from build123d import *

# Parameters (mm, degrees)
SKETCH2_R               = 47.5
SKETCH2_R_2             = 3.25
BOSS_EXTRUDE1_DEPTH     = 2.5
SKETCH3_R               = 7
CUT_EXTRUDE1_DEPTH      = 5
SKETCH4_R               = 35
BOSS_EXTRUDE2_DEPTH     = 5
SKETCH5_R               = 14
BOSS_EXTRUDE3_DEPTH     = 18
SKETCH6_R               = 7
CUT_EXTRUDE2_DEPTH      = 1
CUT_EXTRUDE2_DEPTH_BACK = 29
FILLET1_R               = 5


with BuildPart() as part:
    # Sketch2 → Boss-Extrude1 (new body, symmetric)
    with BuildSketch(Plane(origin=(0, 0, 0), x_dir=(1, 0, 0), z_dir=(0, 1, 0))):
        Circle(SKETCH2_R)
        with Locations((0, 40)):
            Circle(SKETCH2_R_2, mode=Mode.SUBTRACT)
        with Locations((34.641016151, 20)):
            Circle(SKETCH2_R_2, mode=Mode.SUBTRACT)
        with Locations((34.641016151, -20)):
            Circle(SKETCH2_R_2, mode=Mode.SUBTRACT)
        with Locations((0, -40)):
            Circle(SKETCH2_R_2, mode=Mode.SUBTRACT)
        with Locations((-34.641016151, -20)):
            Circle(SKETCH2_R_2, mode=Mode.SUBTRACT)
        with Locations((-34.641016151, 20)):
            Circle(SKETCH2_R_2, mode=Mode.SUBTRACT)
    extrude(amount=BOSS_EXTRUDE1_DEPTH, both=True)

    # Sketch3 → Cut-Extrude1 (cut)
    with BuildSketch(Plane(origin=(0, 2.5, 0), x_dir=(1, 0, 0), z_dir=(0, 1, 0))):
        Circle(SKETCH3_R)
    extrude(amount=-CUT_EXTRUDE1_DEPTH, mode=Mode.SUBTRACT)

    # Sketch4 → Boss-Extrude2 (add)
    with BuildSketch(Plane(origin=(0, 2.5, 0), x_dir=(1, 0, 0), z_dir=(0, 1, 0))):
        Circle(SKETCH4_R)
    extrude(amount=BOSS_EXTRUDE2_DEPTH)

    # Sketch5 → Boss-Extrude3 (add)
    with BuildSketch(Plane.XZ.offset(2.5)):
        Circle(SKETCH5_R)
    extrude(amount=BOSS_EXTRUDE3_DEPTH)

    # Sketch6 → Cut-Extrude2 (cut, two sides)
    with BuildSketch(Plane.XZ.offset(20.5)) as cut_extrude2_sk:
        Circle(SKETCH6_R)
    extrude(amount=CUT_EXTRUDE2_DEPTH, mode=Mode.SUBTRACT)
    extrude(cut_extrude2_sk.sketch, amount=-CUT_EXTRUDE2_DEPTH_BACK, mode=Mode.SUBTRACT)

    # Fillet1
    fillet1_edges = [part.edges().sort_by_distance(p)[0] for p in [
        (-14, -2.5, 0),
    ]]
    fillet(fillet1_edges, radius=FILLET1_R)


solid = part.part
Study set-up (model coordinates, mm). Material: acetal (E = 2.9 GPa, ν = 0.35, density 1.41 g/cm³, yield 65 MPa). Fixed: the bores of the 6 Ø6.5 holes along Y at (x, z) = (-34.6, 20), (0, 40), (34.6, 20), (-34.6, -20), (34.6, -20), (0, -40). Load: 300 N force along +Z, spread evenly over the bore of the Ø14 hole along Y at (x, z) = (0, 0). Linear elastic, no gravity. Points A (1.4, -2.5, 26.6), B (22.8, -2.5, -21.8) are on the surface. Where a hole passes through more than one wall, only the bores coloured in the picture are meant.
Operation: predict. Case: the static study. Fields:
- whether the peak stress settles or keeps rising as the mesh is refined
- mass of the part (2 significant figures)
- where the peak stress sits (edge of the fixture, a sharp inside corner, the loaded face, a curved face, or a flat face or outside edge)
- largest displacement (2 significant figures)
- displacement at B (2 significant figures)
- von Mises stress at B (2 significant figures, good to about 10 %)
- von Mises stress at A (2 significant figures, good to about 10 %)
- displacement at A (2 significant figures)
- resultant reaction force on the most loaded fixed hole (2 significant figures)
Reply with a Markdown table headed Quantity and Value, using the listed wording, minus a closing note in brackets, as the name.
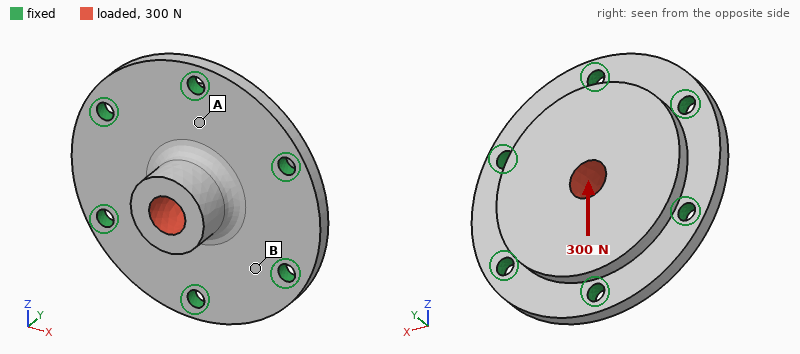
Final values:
| Quantity | Value |
|---|---|
| whether the peak stress settles or keeps rising as the mesh is refined | keeps rising |
| mass of the part | 86 g |
| where the peak stress sits | edge of the fixture |
| largest displacement | 25 µm |
| displacement at B | 4.0 µm |
| von Mises stress at B | 0.27 MPa |
| von Mises stress at A | 0.95 MPa |
| displacement at A | 6.1 µm |
| resultant reaction force on the most loaded fixed hole | 70 N |
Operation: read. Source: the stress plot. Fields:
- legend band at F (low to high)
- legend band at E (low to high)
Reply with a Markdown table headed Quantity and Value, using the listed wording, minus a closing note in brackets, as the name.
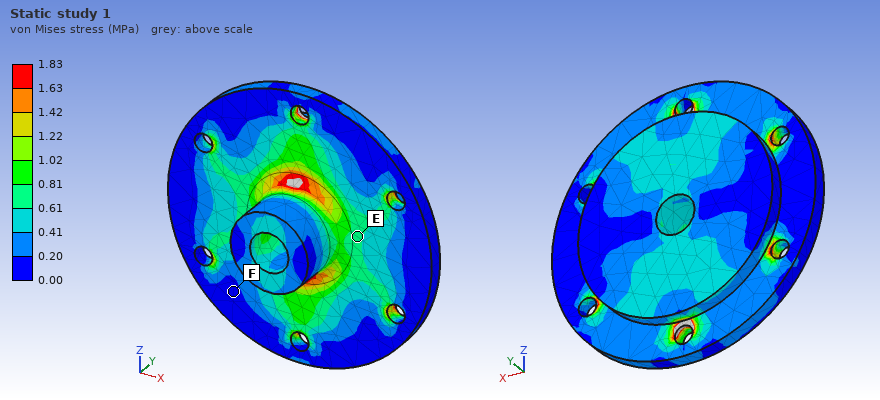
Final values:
| Quantity | Value |
|---|---|
| legend band at F | 0.00 to 0.20 MPa |
| legend band at E | 0.61 to 0.81 MPa |
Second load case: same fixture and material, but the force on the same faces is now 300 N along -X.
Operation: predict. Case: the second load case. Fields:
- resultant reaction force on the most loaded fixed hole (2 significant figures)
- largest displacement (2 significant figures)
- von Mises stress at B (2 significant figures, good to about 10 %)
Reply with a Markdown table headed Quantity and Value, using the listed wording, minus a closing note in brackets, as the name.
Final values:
| Quantity | Value |
|---|---|
| resultant reaction force on the most loaded fixed hole | 63 N |
| largest displacement | 25 µm |
| von Mises stress at B | 0.68 MPa |
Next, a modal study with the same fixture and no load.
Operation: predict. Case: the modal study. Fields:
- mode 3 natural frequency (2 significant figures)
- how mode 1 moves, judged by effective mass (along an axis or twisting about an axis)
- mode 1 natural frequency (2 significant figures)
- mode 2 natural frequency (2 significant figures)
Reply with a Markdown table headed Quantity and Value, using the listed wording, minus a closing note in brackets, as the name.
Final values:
| Quantity | Value |
|---|---|
| mode 3 natural frequency | 3800 Hz |
| how mode 1 moves, judged by effective mass | along Y |
| mode 1 natural frequency | 2500 Hz |
| mode 2 natural frequency | 3800 Hz |
